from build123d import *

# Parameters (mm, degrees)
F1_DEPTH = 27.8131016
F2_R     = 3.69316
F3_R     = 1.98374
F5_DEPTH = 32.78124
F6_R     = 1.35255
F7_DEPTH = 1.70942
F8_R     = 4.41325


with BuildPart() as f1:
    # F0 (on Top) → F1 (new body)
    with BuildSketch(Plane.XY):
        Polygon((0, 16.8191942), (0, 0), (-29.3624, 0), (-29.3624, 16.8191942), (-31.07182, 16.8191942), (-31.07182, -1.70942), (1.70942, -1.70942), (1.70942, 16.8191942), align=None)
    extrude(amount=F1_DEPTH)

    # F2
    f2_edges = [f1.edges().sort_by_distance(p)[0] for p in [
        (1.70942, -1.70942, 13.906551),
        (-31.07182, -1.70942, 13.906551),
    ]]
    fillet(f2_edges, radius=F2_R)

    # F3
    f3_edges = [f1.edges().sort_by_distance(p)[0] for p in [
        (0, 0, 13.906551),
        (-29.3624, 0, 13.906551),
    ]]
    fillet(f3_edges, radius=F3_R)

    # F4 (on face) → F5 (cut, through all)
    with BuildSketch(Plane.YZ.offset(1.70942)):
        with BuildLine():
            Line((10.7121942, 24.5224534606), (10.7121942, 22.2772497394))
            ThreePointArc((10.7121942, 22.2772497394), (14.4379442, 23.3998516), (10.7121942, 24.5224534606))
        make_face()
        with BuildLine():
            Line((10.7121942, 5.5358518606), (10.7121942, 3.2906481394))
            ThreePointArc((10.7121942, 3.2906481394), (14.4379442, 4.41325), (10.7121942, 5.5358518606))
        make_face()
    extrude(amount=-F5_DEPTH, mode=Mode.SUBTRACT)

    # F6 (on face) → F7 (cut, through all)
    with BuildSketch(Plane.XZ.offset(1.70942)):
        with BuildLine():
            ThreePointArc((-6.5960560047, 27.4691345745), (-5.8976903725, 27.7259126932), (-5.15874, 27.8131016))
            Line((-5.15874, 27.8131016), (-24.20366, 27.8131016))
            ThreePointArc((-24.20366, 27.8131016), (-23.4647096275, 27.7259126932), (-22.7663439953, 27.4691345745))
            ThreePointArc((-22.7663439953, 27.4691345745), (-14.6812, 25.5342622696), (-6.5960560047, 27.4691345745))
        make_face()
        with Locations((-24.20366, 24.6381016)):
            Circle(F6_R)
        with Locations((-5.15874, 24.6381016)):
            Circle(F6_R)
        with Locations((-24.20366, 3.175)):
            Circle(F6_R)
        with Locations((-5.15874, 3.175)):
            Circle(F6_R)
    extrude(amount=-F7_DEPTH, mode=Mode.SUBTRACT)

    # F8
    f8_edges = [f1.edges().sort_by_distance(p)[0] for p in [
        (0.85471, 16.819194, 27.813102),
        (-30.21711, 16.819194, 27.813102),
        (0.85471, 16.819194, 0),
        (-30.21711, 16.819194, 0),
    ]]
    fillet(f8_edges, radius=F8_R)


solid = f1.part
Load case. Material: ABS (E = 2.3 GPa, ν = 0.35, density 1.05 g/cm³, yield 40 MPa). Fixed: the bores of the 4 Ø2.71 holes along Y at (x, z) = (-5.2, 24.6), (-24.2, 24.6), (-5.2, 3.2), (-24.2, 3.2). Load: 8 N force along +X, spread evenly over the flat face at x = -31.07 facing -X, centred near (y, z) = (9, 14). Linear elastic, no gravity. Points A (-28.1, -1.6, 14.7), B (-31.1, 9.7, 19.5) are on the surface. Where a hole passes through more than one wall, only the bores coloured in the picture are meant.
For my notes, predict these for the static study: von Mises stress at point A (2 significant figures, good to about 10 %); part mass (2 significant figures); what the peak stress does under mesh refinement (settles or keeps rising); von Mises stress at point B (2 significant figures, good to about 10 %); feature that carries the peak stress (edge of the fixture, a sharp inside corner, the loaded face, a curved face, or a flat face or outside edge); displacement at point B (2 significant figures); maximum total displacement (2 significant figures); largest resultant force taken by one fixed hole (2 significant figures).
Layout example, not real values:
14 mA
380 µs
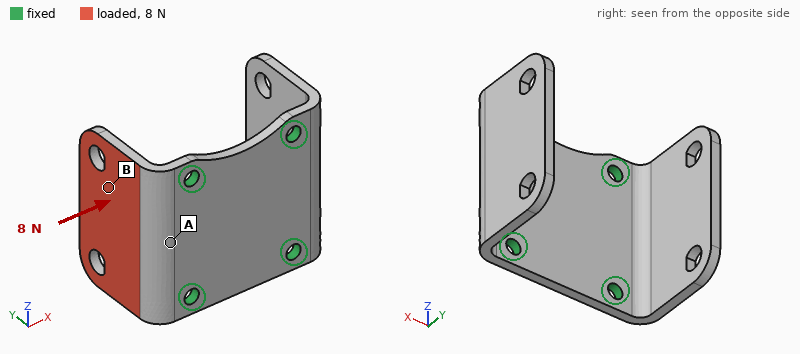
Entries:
3.6 MPa
3.0 g
keeps rising
0.99 MPa
edge of the fixture
0.25 mm
0.46 mm
3.0 N
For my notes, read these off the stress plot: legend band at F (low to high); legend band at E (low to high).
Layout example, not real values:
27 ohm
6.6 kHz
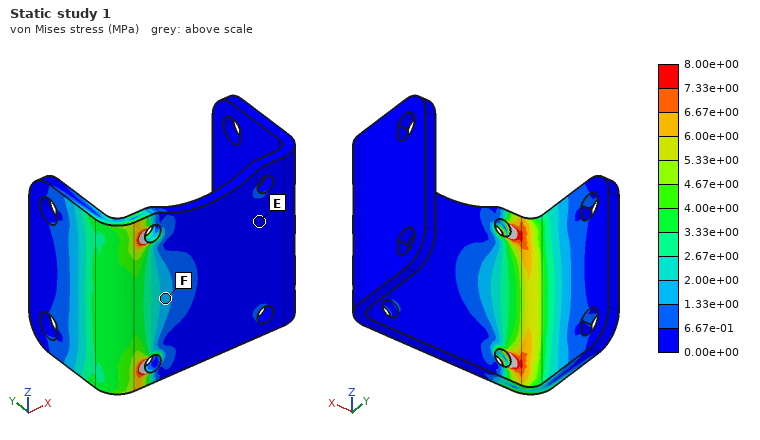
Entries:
1.33e+00 to 2.00e+00 MPa
0.00e+00 to 6.67e-01 MPa
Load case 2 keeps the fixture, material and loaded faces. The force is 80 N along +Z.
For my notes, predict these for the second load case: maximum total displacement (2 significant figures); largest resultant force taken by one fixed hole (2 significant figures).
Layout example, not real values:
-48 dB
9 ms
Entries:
0.30 mm
58 N
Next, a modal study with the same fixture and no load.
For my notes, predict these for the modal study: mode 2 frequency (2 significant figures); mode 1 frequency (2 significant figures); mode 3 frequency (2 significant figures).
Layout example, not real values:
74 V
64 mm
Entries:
1000 Hz
990 Hz
2100 Hz
